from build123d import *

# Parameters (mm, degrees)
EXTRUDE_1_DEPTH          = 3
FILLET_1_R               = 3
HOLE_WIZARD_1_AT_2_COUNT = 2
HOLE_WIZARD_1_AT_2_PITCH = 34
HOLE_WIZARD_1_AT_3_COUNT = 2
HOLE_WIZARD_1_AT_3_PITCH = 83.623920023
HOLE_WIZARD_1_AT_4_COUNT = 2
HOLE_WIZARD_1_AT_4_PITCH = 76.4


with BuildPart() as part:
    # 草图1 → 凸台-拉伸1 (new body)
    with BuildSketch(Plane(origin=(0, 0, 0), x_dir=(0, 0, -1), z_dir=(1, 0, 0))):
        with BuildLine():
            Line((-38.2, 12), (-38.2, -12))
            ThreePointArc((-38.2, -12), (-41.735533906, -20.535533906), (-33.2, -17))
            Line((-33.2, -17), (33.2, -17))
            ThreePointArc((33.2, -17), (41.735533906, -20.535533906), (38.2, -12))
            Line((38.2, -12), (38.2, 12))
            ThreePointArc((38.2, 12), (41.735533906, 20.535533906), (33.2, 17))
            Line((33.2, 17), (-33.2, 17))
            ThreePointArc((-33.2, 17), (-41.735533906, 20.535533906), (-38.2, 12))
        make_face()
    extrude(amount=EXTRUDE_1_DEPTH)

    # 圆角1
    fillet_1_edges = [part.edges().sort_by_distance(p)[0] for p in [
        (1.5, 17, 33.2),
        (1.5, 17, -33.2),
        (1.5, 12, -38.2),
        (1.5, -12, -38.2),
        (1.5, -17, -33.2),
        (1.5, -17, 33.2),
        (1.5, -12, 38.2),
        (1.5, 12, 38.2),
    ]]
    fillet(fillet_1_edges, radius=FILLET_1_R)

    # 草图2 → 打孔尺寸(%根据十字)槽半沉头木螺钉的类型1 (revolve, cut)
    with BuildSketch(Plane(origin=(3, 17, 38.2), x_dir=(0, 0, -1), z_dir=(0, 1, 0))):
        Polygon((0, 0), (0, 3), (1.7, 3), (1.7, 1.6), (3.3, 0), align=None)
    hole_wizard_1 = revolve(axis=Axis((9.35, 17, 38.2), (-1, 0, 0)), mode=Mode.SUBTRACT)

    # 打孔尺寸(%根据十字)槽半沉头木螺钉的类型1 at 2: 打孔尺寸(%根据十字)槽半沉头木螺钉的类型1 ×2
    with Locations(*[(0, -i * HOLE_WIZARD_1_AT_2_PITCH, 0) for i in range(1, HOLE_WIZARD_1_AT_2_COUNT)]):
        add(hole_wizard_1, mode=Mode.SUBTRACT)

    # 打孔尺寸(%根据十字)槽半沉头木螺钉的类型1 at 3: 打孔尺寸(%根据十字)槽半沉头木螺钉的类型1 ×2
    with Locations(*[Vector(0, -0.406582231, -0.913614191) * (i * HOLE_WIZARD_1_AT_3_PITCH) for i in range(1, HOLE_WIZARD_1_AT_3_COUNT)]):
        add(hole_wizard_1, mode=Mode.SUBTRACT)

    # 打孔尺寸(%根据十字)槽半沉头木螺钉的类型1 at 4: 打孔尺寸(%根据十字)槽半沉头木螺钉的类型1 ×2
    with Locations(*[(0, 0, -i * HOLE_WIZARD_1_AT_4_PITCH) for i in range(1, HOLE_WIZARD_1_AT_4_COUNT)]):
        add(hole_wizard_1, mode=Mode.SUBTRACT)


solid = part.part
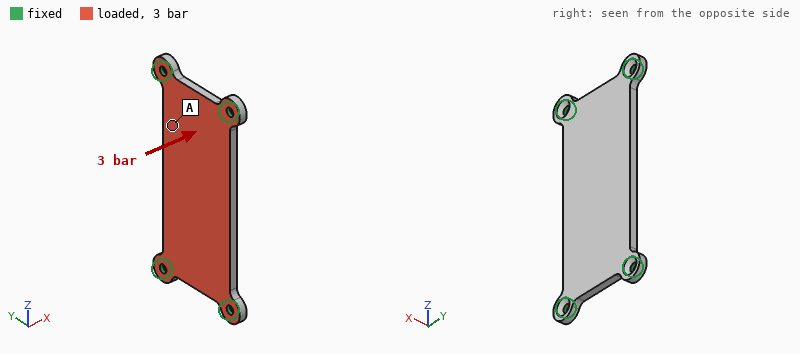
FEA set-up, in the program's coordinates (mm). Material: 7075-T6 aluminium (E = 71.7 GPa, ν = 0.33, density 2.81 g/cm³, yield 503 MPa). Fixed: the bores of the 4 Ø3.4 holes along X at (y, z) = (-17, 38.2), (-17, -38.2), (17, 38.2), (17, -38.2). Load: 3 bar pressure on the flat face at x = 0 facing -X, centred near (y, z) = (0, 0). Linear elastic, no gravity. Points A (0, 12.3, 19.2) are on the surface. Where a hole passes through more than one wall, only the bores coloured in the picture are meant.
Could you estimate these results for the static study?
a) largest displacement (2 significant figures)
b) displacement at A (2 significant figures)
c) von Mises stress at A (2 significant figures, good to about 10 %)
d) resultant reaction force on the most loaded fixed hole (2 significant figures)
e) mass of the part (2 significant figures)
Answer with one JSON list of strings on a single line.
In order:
["0.28 mm", "0.17 mm", "31 MPa", "350 N", "23 g"]
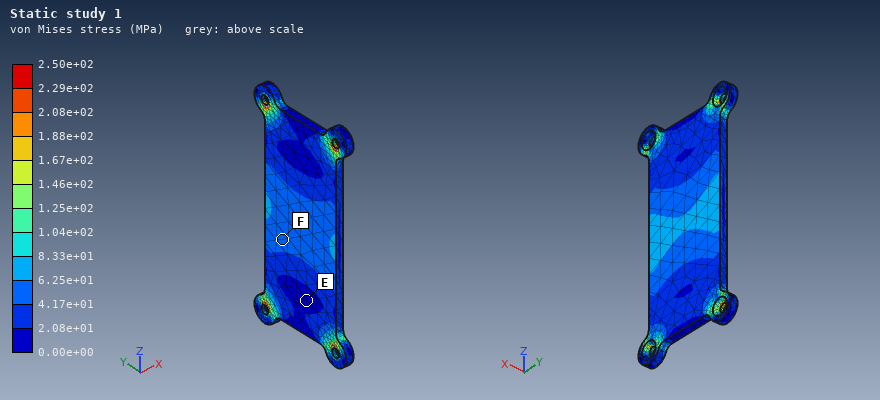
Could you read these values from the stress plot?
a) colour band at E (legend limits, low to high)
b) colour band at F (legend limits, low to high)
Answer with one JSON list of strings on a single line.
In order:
["0.00e+00 to 2.08e+01 MPa", "4.17e+01 to 6.25e+01 MPa"]
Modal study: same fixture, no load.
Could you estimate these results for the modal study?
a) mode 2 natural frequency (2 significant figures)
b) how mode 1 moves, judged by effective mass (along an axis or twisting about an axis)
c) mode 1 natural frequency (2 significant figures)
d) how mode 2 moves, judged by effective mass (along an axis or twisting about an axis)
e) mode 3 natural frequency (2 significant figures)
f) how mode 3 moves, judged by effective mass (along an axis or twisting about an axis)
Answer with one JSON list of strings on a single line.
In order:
["4500 Hz", "along X", "2100 Hz", "twisting about Z", "5800 Hz", "twisting about Y"]
